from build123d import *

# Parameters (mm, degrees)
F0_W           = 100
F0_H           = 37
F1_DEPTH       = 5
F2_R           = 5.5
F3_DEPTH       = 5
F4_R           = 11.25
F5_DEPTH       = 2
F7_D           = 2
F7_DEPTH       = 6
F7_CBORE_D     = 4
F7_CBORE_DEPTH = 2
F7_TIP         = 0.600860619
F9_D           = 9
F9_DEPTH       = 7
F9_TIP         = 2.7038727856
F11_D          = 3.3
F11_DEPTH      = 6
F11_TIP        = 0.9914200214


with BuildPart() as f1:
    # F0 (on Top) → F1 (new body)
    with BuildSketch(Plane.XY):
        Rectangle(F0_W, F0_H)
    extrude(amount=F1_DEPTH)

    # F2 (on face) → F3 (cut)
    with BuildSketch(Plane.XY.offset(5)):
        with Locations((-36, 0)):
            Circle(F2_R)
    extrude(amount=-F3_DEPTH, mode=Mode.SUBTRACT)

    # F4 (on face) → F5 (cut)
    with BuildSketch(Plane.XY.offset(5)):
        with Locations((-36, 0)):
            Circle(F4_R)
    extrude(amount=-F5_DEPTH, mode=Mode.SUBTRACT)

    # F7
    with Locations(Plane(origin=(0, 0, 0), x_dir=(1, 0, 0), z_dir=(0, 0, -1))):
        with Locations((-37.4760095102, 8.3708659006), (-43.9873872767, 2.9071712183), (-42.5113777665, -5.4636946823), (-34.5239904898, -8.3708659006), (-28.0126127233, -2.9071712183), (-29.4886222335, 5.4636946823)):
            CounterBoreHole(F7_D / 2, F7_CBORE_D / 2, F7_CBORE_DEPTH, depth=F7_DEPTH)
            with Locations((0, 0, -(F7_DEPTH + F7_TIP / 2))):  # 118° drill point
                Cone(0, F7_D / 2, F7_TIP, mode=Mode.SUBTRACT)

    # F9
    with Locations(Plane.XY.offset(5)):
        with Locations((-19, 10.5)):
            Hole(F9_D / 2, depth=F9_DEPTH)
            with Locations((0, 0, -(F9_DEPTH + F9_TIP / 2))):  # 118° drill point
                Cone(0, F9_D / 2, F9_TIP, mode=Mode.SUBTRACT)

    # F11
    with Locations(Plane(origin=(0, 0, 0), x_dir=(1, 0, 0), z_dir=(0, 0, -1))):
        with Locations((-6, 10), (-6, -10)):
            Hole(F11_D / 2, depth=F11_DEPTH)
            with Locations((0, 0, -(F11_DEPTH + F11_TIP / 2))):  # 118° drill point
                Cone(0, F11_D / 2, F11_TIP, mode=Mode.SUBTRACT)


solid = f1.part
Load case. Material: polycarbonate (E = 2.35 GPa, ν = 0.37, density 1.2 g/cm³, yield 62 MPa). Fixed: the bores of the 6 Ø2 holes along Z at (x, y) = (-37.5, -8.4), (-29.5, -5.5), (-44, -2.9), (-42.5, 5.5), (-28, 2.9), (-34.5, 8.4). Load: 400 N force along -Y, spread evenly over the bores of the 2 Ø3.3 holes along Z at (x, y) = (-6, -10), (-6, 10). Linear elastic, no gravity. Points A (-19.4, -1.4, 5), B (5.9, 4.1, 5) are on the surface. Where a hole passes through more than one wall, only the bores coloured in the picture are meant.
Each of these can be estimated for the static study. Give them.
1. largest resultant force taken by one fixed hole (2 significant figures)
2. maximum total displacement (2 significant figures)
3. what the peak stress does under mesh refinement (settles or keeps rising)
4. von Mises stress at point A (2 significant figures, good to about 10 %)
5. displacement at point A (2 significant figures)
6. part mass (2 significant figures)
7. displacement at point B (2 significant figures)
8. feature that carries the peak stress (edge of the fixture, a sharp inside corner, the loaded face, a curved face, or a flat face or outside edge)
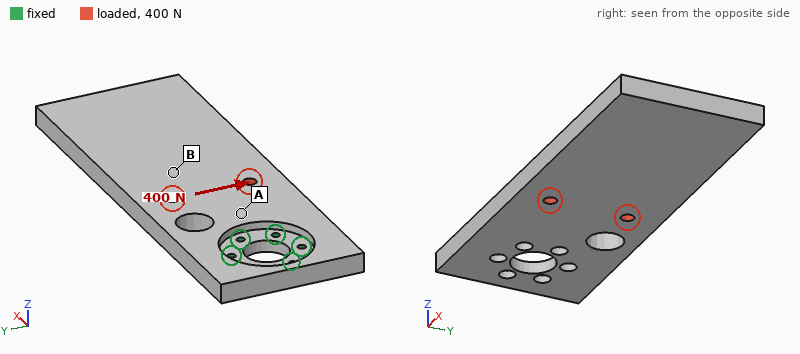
320 N
0.84 mm
keeps rising
7.9 MPa
0.14 mm
20 g
0.42 mm
edge of the fixture
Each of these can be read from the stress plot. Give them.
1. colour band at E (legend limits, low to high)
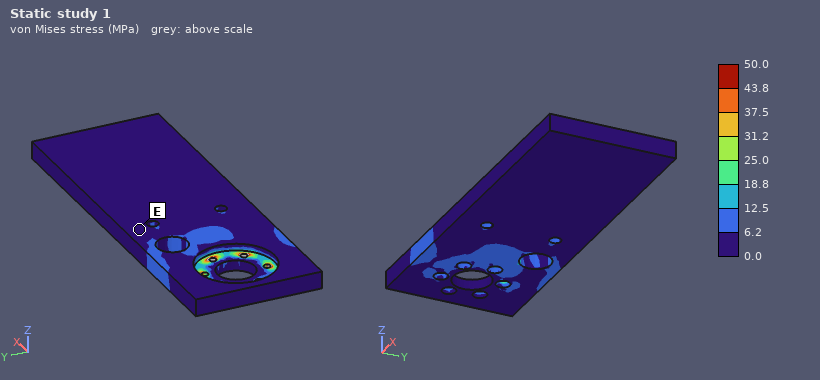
0.0 to 6.2 MPa
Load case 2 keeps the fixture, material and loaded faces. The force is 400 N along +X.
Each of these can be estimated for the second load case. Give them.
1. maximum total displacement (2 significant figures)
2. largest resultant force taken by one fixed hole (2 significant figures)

0.20 mm
110 N
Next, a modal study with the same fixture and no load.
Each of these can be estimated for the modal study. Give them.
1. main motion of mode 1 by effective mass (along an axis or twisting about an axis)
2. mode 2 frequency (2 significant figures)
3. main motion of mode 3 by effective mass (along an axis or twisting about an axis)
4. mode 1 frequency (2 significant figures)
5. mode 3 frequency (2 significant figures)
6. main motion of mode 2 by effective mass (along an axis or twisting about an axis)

along Z
590 Hz
along Y
130 Hz
720 Hz
twisting about X
